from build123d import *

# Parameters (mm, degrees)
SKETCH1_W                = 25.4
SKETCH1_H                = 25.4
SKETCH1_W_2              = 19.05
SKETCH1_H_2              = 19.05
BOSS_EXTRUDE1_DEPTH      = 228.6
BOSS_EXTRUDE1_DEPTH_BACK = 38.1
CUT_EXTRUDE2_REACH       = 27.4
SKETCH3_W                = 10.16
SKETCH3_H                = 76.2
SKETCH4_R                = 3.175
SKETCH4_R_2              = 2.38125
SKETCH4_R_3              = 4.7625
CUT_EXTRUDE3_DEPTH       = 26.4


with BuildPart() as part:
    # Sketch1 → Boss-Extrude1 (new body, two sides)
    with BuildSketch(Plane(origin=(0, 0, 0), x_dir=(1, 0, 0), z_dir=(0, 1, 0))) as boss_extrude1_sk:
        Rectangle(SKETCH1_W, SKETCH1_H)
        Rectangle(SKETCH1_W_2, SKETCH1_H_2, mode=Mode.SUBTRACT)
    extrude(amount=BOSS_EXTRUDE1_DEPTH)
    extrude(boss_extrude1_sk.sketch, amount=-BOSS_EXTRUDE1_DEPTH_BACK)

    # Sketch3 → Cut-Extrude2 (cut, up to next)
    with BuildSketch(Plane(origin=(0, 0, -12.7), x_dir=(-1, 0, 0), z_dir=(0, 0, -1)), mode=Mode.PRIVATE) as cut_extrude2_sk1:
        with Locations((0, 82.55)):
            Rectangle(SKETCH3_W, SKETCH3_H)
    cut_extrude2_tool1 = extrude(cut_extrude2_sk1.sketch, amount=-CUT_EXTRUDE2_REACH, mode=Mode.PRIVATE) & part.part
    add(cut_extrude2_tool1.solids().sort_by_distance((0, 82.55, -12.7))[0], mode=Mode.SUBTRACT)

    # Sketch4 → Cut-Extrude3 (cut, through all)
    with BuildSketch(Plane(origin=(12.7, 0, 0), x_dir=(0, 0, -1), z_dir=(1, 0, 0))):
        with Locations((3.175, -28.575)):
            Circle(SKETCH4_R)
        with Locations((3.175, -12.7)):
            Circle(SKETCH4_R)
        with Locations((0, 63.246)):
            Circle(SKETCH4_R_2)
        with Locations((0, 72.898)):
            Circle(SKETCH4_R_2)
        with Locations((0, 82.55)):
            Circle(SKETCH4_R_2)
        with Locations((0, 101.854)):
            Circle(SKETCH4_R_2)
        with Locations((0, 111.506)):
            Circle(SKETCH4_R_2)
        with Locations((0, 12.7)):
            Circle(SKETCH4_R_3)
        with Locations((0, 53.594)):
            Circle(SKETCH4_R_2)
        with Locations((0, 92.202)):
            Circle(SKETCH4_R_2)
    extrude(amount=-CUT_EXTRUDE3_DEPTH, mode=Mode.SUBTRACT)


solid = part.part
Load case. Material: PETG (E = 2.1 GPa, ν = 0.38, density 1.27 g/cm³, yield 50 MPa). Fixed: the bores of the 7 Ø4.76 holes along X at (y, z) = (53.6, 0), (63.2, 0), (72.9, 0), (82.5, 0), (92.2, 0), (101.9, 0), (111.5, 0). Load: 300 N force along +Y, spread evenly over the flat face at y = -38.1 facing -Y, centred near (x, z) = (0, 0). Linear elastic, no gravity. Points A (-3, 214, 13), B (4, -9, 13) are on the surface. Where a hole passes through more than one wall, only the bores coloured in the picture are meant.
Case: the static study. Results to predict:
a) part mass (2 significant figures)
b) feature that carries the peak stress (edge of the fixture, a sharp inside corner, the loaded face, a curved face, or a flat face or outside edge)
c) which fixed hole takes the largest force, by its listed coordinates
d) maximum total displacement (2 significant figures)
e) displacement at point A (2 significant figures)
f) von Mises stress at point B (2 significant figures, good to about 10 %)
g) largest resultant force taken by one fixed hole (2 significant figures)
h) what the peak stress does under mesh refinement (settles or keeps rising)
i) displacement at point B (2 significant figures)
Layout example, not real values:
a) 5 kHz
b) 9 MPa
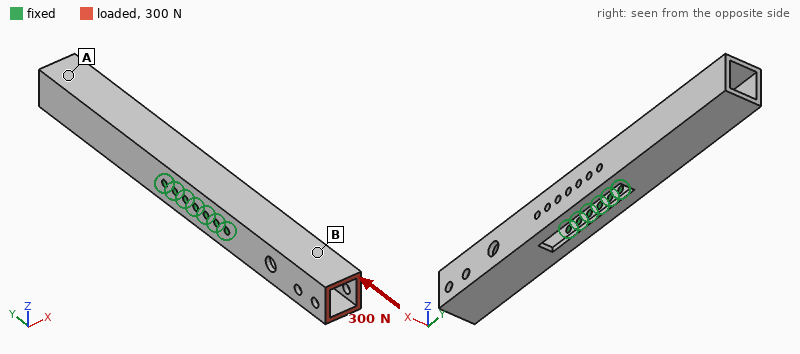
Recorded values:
a) 90 g
b) edge of the fixture
c) (53.6, 0)
d) 0.59 mm
e) 0.51 mm
f) 1.2 MPa
g) 120 N
h) keeps rising
i) 0.40 mm
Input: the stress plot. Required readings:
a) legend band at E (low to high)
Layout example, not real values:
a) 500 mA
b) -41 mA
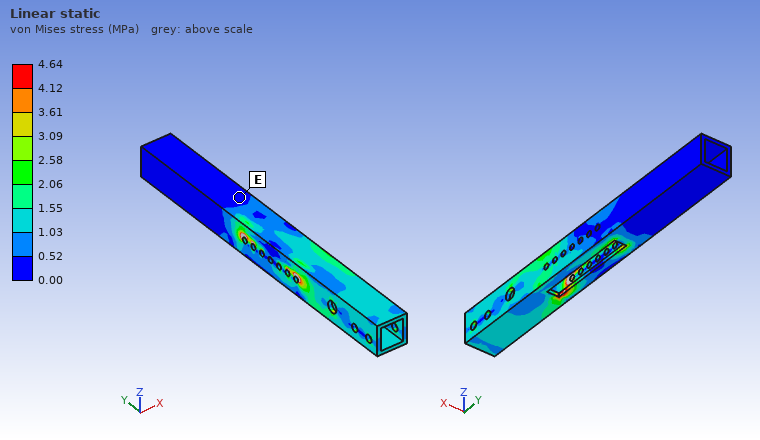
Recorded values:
a) 0.00 to 0.52 MPa
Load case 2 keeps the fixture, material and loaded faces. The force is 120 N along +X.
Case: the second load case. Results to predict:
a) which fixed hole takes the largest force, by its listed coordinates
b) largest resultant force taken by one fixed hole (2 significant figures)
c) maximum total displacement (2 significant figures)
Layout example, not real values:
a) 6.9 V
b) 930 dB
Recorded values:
a) (53.6, 0)
b) 360 N
c) 2.8 mm
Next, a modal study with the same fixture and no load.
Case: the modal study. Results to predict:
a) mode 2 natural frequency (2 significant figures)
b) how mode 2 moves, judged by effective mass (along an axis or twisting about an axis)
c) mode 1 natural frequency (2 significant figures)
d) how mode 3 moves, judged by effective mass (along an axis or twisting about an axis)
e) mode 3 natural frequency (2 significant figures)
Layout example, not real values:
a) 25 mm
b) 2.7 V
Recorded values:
a) 270 Hz
b) along Z
c) 200 Hz
d) along Z
e) 340 Hz
